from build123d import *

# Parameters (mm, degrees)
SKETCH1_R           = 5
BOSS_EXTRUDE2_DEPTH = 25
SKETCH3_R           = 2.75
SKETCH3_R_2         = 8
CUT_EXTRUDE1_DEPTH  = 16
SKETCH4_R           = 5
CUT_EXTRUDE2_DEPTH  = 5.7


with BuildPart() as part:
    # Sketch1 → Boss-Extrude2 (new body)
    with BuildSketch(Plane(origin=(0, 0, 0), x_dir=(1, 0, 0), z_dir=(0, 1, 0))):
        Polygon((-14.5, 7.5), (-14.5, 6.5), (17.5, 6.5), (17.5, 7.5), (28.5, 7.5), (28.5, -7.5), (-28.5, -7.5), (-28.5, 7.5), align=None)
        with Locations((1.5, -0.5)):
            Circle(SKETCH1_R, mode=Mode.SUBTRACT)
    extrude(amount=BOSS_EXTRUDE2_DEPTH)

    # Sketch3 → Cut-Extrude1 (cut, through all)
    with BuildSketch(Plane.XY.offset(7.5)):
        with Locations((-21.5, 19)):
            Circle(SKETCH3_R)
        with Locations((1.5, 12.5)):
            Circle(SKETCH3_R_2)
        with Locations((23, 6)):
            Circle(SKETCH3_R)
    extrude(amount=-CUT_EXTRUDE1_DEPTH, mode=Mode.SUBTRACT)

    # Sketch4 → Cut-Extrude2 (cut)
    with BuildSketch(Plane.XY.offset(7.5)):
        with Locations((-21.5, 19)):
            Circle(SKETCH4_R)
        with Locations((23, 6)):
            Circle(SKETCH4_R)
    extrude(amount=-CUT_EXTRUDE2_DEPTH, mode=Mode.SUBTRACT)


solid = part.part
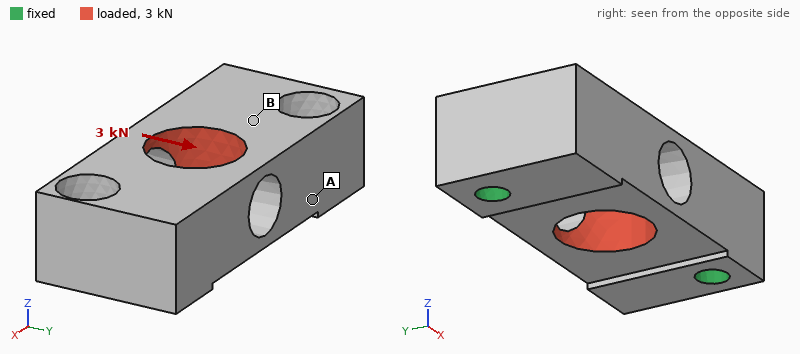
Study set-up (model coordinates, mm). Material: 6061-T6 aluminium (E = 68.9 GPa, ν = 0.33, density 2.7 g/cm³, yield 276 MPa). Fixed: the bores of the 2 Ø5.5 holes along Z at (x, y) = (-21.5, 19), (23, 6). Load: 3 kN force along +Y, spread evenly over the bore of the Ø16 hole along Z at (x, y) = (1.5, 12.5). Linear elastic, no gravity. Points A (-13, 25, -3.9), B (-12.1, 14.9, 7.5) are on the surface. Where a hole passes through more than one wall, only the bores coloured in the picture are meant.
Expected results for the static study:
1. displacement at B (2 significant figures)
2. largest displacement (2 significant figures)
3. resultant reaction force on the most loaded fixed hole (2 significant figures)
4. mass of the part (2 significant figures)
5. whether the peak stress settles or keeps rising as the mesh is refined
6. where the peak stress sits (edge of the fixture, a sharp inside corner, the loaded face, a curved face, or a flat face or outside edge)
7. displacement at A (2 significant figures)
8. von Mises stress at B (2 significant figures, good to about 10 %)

8.5 µm
16 µm
1.5 kN
42 g
keeps rising
edge of the fixture
5.4 µm
13 MPa
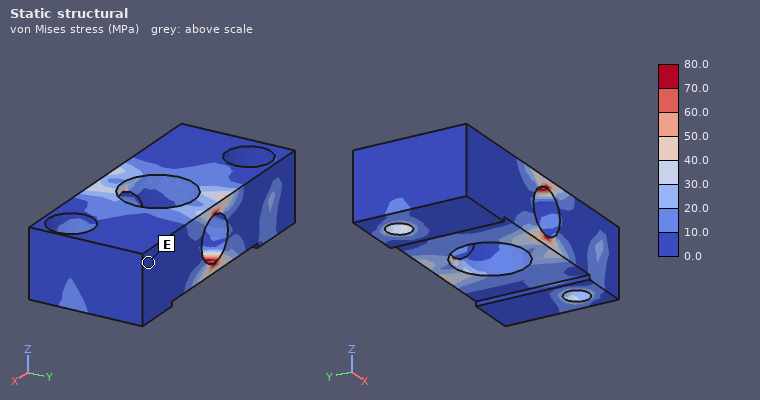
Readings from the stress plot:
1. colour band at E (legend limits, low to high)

0.0 to 10.0 MPa
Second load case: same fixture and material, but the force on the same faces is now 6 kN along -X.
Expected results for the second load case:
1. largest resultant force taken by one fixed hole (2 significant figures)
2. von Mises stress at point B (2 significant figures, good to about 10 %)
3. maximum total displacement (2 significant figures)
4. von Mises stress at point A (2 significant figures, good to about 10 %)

3.0 kN
11 MPa
12 µm
14 MPa
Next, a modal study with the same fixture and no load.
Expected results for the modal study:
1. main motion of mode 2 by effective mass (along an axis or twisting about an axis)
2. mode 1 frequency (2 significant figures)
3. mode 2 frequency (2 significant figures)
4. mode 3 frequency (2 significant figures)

along Z
14 kHz
15 kHz
18 kHz
